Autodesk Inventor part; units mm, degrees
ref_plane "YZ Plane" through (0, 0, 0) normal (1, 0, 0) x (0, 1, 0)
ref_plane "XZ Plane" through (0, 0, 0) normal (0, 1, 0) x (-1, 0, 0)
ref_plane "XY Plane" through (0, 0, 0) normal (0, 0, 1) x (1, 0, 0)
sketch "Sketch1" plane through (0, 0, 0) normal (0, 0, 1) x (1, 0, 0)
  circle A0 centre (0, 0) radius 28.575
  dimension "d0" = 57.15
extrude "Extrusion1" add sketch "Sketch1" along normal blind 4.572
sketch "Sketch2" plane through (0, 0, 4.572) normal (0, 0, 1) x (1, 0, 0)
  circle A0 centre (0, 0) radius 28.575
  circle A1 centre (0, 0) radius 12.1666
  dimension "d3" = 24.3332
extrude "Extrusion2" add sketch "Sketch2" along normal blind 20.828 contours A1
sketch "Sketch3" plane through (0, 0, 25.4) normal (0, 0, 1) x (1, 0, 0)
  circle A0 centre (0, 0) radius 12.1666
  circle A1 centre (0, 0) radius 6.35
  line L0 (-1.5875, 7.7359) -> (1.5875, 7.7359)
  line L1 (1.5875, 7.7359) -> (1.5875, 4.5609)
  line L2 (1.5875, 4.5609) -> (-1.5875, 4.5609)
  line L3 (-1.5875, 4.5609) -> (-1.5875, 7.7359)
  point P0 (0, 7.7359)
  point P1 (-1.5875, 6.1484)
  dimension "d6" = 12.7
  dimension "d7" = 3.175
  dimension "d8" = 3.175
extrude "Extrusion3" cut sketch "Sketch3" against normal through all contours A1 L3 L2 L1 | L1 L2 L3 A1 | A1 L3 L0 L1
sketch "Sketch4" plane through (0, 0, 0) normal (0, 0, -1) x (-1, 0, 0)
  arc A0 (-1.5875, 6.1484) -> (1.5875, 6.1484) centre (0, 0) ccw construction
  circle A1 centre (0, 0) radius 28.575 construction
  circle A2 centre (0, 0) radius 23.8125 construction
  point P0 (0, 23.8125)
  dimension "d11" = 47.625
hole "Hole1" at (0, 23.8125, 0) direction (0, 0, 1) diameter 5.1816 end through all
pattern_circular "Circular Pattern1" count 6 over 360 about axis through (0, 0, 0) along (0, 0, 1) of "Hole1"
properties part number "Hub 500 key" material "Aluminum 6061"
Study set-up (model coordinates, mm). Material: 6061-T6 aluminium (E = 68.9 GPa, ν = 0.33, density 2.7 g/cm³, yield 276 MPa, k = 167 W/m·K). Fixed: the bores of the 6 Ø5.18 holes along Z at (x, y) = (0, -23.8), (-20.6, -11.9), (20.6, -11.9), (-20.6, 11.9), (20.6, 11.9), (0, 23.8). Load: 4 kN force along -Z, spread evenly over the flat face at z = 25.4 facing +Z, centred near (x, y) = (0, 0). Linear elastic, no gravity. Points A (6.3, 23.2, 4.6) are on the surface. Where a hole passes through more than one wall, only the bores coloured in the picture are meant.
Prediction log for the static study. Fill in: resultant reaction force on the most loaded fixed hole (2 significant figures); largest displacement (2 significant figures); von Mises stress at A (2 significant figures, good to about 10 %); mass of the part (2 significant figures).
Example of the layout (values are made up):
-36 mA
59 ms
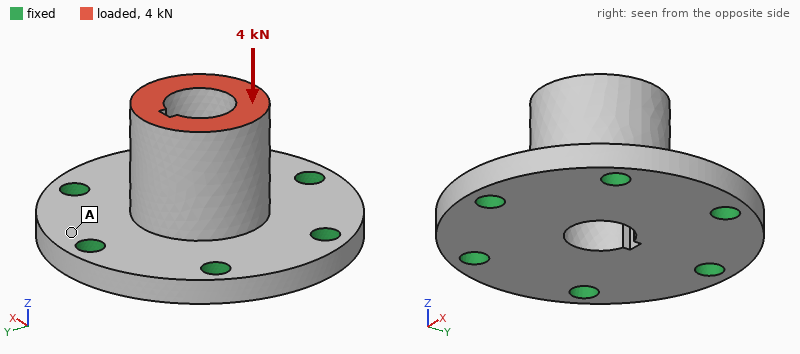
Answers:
740 N
24 µm
17 MPa
47 g
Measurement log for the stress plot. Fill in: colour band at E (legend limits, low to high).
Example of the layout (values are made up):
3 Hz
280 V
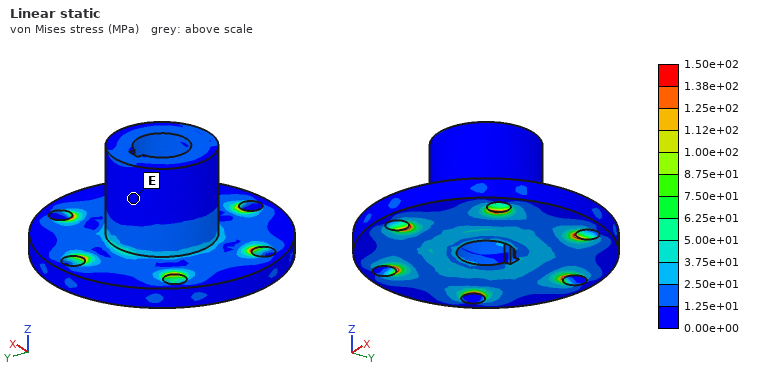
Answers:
0.00e+00 to 1.25e+01 MPa
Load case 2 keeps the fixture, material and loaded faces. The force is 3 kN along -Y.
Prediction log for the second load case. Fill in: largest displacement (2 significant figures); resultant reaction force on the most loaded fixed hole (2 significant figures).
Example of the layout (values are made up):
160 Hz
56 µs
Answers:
79 µm
1.5 kN
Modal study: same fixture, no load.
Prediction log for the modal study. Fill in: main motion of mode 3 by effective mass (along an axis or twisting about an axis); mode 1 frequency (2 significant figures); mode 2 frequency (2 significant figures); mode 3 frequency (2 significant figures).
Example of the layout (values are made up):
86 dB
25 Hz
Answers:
along Z
12 kHz
12 kHz
14 kHz
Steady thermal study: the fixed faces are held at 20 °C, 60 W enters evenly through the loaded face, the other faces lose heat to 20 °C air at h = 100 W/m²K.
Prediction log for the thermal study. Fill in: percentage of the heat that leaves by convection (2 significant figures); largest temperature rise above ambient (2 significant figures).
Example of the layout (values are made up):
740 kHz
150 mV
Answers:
12 %
32 K
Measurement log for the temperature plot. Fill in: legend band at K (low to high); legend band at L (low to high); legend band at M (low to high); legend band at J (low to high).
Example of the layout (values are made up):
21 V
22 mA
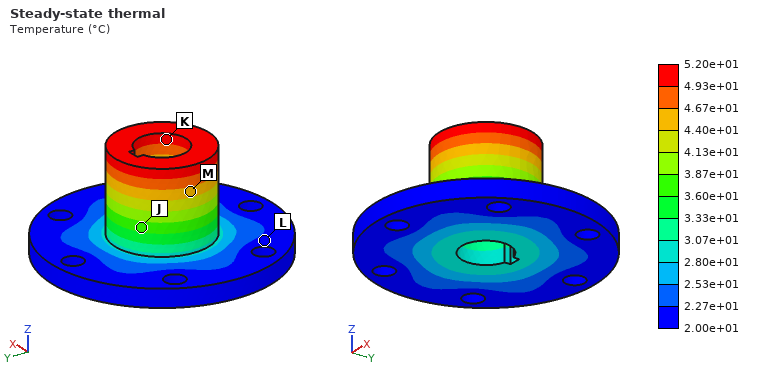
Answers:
4.93e+01 to 5.20e+01 °C
2.00e+01 to 2.27e+01 °C
4.40e+01 to 4.67e+01 °C
3.60e+01 to 3.87e+01 °C
